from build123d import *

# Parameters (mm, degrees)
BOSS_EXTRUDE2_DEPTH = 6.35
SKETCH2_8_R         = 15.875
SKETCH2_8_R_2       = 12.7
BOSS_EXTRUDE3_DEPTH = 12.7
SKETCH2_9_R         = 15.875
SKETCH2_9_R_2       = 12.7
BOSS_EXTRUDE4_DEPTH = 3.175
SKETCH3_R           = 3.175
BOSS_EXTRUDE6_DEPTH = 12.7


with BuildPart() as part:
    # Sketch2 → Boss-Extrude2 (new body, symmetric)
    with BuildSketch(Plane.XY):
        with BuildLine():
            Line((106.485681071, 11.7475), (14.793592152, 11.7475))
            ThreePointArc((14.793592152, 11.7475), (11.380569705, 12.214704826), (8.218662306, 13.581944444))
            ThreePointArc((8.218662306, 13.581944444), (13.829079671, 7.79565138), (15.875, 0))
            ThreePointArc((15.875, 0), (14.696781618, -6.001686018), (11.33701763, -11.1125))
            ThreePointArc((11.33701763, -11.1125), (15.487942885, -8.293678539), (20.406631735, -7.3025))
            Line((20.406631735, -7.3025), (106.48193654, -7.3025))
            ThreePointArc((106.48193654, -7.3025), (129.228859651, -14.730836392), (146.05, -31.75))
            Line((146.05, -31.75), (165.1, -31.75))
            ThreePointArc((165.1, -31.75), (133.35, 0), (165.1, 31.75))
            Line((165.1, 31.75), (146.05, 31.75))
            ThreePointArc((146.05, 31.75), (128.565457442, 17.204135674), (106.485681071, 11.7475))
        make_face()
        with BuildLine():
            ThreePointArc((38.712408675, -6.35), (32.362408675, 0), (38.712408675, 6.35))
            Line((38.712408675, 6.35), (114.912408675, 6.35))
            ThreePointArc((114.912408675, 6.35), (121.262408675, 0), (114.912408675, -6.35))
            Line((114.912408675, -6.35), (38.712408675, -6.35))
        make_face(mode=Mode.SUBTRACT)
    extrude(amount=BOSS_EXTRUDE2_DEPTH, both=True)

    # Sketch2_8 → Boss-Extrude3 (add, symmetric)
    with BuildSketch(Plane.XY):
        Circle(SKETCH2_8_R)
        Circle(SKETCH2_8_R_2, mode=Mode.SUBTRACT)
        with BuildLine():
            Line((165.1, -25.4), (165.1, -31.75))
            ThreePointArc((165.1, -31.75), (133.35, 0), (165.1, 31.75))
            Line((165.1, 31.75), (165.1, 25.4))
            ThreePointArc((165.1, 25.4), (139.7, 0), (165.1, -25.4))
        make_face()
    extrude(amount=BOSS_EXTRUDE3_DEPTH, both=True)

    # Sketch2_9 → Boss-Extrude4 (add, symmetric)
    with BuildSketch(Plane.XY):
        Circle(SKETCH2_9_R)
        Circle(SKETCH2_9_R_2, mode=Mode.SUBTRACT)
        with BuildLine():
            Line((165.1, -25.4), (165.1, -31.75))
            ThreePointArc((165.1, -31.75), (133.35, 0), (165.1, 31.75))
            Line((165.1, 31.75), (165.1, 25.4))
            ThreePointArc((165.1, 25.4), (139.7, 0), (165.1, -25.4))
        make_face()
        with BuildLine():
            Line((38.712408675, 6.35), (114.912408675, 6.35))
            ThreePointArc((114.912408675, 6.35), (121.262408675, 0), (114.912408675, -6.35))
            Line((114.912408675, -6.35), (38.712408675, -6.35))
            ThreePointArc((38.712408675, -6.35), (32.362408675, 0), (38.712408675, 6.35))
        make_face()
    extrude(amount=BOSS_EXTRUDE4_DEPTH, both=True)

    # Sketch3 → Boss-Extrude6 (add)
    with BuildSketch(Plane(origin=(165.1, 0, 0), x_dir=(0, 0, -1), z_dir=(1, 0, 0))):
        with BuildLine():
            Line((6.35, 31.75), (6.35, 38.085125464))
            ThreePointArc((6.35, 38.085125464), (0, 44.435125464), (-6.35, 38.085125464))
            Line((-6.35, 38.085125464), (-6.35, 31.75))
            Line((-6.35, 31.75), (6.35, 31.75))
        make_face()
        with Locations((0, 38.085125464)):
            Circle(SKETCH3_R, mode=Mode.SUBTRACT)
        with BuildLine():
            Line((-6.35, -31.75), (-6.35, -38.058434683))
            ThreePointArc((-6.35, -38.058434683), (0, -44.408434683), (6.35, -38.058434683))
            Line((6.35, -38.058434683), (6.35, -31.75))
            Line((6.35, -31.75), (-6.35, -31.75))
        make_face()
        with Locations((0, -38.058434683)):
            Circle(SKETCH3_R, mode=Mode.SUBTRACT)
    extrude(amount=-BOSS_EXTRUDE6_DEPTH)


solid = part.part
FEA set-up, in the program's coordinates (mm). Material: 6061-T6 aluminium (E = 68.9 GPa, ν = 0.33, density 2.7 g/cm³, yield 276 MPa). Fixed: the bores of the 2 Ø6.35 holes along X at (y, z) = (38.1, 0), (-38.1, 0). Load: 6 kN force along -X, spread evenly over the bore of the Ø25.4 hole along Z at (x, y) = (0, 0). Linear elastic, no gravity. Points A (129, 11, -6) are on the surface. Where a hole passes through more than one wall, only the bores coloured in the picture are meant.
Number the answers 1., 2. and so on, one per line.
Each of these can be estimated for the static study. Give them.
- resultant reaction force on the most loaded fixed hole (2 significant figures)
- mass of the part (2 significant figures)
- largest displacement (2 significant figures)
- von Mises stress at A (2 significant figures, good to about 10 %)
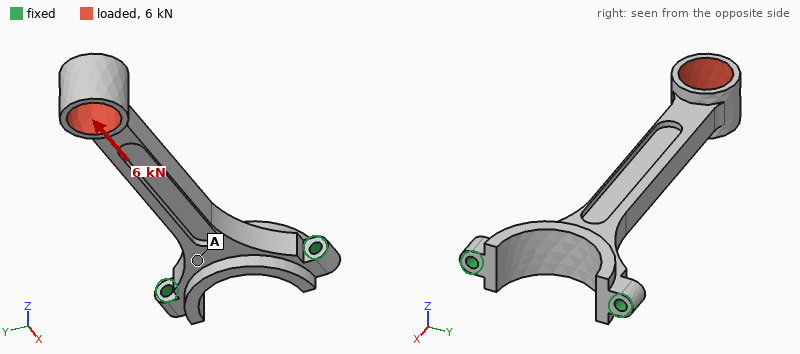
1. 3.9 kN
2. 140 g
3. 0.54 mm
4. 18 MPa
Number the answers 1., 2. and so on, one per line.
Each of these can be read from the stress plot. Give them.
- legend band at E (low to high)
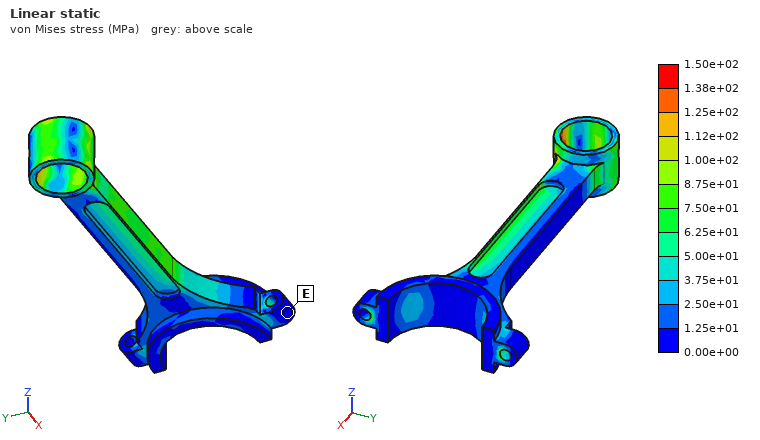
1. 0.00e+00 to 1.25e+01 MPa
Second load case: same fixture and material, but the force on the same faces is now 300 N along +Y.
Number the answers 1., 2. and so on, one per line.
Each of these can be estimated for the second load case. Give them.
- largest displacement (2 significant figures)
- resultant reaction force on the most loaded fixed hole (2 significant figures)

1. 0.66 mm
2. 900 N
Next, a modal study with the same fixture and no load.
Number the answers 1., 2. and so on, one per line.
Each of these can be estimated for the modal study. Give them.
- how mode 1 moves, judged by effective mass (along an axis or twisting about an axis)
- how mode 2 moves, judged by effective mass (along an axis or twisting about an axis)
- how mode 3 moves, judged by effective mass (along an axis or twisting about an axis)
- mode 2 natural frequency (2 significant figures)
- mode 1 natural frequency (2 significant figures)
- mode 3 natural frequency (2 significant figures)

1. along Z
2. along Y
3. along Z
4. 680 Hz
5. 300 Hz
6. 1700 Hz
